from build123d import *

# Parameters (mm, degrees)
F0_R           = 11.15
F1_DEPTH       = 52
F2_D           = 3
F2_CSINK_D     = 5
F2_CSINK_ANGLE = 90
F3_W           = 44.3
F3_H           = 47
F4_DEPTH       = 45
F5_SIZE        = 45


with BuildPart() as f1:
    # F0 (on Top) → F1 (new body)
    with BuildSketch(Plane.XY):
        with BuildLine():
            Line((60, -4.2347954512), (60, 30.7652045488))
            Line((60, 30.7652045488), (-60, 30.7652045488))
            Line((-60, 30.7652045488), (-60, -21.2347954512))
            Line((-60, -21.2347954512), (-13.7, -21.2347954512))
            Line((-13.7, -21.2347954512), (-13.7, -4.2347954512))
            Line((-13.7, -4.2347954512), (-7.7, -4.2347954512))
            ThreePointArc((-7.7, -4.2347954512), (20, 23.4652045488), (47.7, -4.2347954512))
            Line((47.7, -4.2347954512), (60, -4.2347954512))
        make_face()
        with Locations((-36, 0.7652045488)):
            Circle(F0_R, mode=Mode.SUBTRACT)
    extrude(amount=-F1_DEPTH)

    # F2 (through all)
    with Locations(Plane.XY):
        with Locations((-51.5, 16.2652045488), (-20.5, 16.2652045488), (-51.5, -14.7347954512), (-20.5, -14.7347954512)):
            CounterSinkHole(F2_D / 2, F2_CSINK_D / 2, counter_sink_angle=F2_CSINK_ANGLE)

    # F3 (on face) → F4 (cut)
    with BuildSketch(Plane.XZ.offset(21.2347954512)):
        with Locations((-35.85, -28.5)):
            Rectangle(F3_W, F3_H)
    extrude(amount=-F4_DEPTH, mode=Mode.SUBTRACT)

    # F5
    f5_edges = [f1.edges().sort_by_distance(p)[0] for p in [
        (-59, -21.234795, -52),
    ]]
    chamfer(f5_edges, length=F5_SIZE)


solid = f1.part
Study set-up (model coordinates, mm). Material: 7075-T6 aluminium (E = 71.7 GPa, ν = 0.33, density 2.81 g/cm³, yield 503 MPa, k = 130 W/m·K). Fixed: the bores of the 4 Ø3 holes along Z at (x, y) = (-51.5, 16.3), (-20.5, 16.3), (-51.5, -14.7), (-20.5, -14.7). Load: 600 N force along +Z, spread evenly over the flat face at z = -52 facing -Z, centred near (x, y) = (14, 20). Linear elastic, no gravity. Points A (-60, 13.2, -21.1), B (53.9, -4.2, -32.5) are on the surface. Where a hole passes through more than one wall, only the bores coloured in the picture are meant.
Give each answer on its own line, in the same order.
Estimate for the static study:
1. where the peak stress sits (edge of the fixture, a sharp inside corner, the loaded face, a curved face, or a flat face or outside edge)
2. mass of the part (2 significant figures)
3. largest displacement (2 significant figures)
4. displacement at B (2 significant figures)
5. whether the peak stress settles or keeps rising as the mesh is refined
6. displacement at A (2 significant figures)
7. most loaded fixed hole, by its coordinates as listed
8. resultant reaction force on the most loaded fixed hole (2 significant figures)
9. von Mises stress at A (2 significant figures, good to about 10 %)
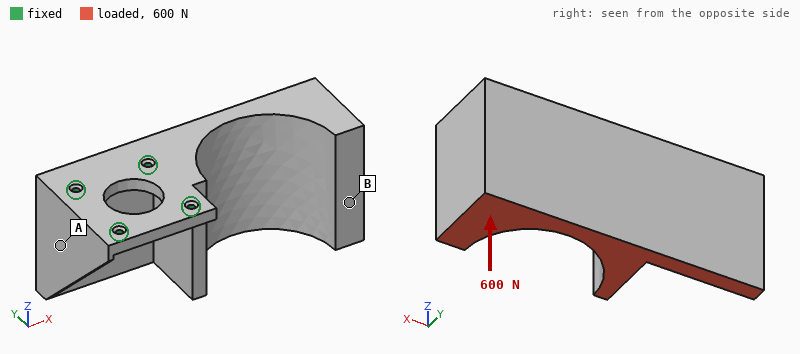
edge of the fixture
280 g
92 µm
70 µm
keeps rising
16 µm
(-20.5, 16.3)
1.2 kN
5.8 MPa
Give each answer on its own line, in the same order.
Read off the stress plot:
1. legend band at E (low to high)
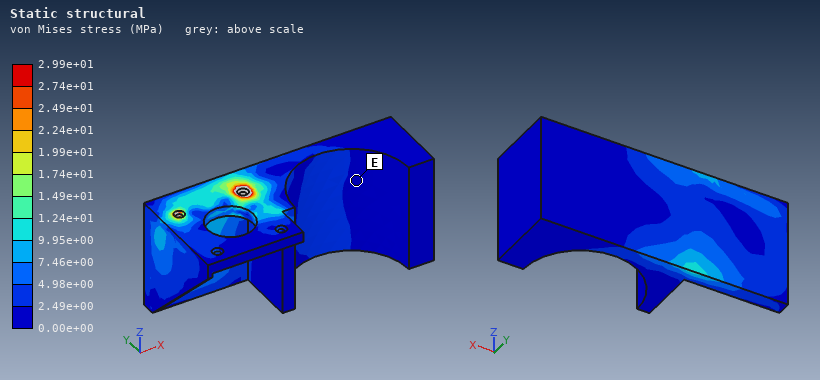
0.00e+00 to 2.49e+00 MPa
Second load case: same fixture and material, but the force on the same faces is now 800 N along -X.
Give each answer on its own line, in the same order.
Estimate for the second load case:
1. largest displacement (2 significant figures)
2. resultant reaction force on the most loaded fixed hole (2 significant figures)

0.15 mm
1.3 kN
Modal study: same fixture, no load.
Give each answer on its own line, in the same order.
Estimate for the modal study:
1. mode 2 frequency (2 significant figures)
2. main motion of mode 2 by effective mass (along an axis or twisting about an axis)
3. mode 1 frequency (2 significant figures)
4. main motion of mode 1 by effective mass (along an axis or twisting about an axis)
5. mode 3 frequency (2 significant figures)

1000 Hz
along Z
720 Hz
along Y
1700 Hz
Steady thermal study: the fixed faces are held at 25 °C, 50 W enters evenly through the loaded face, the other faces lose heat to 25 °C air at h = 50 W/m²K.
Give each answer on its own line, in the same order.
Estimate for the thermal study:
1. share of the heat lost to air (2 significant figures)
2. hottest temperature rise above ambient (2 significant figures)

42 %
33 K
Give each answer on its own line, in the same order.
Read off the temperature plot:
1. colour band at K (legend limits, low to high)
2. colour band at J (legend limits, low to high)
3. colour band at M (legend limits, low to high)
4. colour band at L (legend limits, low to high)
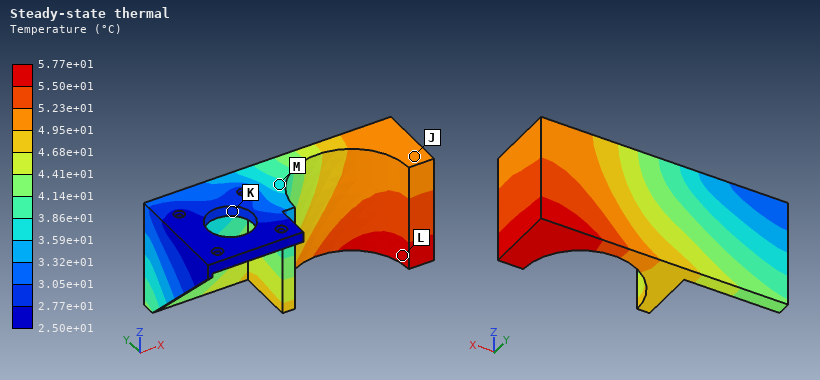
2.77e+01 to 3.05e+01 °C
4.95e+01 to 5.23e+01 °C
3.59e+01 to 3.86e+01 °C
5.50e+01 to 5.77e+01 °C
